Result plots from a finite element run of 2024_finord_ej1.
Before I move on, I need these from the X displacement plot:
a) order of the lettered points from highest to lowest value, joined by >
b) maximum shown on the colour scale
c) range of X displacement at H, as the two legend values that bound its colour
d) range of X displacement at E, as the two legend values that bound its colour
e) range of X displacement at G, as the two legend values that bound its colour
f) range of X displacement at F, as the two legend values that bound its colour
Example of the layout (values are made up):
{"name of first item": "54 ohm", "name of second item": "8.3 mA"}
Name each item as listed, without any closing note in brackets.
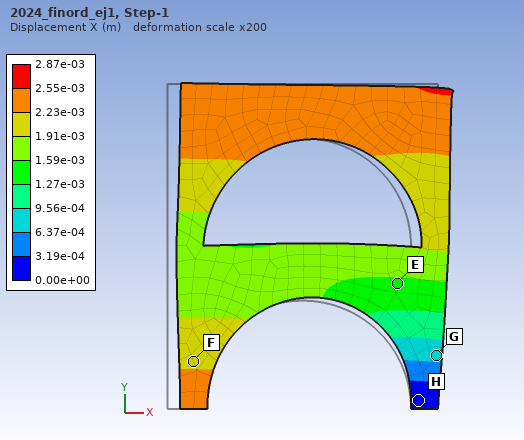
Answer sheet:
{"order of the lettered points from highest to lowest value, joined by >": "F > E > G > H", "maximum shown on the colour scale": "2.87e-03 m", "range of X displacement at H, as the two legend values that bound its colour": "0.00e+00 to 3.19e-04 m", "range of X displacement at E, as the two legend values that bound its colour": "1.27e-03 to 1.59e-03 m", "range of X displacement at G, as the two legend values that bound its colour": "6.37e-04 to 9.56e-04 m", "range of X displacement at F, as the two legend values that bound its colour": "1.91e-03 to 2.23e-03 m"}
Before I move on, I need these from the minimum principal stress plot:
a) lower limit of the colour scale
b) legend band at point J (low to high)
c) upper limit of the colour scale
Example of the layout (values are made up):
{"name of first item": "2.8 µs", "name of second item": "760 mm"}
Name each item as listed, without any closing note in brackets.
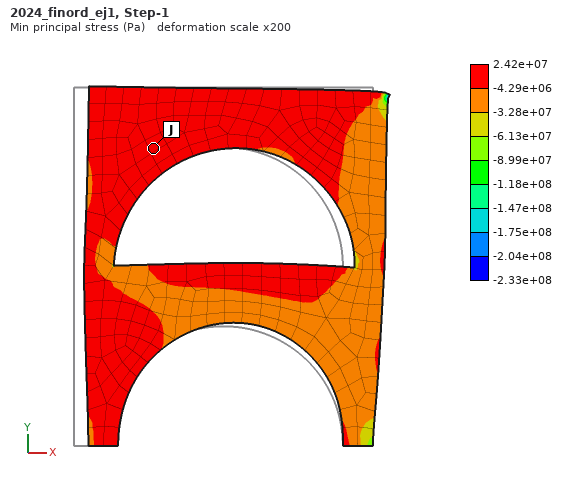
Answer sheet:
{"lower limit of the colour scale": "-2.33e+08 Pa", "legend band at point J": "-4.29e+06 to 2.42e+07 Pa", "upper limit of the colour scale": "2.42e+07 Pa"}
